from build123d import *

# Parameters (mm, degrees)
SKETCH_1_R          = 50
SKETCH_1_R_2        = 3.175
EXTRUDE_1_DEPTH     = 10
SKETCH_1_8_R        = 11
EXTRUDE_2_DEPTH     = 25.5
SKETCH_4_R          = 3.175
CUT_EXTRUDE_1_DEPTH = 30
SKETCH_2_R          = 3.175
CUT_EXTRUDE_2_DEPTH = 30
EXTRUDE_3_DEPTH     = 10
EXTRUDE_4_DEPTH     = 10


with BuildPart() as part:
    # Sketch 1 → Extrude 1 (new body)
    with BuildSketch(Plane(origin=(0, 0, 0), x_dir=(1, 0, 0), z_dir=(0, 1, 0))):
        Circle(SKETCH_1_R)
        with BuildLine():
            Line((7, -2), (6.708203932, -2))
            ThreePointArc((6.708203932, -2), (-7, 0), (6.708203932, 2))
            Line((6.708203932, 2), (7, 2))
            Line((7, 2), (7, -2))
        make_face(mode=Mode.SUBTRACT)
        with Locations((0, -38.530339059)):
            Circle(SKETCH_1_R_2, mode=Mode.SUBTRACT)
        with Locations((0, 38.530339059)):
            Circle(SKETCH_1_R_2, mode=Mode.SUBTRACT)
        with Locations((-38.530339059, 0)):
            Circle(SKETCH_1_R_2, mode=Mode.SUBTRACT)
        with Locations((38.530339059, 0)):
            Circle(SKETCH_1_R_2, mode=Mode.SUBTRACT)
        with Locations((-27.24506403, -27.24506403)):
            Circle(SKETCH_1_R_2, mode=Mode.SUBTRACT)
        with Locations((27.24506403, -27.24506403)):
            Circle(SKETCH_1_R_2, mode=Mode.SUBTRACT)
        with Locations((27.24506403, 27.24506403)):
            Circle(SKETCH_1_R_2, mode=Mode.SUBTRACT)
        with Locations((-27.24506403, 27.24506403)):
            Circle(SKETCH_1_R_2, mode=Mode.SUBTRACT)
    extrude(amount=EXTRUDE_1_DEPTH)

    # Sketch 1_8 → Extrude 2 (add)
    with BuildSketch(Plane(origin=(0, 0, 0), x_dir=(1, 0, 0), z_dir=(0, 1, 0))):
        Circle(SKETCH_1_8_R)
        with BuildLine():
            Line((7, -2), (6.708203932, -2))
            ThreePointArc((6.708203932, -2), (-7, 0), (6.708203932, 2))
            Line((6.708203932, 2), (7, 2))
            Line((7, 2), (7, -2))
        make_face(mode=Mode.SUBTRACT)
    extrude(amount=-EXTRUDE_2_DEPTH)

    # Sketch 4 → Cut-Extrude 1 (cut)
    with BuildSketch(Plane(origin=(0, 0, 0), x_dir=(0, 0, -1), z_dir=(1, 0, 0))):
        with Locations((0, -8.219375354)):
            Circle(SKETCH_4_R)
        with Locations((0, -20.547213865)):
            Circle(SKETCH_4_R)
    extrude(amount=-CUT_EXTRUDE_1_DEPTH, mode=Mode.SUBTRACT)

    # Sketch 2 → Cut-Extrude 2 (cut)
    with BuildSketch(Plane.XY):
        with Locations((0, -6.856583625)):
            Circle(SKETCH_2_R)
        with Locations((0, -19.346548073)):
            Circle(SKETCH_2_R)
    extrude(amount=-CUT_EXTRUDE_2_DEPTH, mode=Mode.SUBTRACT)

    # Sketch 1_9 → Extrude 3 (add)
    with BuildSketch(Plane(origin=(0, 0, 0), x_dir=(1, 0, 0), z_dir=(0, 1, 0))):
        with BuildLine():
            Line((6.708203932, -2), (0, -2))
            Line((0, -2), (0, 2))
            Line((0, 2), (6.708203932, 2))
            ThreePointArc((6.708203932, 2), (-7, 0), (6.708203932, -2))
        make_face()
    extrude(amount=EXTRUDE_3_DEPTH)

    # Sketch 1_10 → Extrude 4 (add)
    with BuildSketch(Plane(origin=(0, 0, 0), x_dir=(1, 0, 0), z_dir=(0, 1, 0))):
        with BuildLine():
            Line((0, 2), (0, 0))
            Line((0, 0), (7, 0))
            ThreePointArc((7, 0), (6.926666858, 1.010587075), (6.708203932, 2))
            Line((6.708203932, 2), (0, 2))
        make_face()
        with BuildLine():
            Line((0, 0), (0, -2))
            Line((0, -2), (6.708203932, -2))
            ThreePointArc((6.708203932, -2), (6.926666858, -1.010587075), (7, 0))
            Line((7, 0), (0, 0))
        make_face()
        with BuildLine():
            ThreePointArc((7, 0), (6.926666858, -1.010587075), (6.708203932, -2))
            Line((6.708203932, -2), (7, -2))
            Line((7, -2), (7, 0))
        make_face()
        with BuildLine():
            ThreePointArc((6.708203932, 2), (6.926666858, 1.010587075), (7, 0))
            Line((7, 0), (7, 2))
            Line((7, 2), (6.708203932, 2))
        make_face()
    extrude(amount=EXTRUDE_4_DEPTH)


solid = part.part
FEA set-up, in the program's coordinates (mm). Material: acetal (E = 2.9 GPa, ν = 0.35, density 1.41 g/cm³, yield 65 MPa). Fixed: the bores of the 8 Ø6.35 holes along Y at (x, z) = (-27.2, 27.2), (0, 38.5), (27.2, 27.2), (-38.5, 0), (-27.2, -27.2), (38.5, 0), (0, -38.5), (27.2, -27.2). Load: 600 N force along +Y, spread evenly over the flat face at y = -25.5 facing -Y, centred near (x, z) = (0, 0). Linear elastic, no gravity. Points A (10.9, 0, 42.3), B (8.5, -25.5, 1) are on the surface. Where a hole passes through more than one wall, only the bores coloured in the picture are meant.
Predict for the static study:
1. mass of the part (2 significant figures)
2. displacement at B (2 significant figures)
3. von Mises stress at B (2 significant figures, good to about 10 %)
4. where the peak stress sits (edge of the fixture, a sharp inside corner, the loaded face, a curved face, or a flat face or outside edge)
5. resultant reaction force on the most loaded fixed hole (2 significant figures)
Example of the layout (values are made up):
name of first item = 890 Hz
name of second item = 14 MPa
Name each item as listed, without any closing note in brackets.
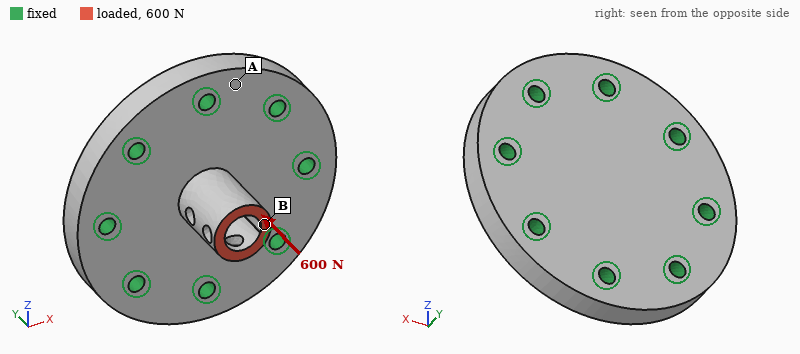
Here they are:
mass of the part = 110 g
displacement at B = 0.076 mm
von Mises stress at B = 2.7 MPa
where the peak stress sits = a curved face
resultant reaction force on the most loaded fixed hole = 77 N
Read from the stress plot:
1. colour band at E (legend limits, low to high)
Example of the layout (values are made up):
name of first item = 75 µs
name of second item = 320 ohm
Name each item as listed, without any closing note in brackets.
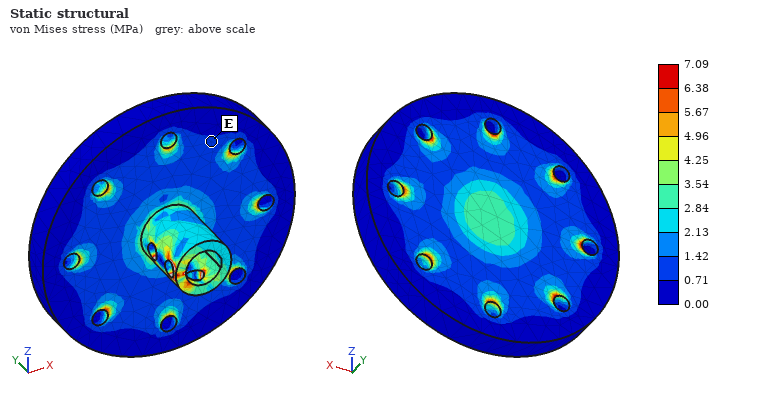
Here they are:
colour band at E = 0.71 to 1.42 MPa
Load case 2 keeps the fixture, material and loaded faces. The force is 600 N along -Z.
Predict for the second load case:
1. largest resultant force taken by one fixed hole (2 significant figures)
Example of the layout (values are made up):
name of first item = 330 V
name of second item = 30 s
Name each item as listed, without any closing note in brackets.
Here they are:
largest resultant force taken by one fixed hole = 210 N
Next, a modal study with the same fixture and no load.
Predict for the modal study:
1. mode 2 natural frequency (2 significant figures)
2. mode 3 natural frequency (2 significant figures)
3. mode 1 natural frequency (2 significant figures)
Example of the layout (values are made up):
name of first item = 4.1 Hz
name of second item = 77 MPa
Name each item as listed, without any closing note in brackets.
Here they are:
mode 2 natural frequency = 3400 Hz
mode 3 natural frequency = 3400 Hz
mode 1 natural frequency = 3400 Hz
